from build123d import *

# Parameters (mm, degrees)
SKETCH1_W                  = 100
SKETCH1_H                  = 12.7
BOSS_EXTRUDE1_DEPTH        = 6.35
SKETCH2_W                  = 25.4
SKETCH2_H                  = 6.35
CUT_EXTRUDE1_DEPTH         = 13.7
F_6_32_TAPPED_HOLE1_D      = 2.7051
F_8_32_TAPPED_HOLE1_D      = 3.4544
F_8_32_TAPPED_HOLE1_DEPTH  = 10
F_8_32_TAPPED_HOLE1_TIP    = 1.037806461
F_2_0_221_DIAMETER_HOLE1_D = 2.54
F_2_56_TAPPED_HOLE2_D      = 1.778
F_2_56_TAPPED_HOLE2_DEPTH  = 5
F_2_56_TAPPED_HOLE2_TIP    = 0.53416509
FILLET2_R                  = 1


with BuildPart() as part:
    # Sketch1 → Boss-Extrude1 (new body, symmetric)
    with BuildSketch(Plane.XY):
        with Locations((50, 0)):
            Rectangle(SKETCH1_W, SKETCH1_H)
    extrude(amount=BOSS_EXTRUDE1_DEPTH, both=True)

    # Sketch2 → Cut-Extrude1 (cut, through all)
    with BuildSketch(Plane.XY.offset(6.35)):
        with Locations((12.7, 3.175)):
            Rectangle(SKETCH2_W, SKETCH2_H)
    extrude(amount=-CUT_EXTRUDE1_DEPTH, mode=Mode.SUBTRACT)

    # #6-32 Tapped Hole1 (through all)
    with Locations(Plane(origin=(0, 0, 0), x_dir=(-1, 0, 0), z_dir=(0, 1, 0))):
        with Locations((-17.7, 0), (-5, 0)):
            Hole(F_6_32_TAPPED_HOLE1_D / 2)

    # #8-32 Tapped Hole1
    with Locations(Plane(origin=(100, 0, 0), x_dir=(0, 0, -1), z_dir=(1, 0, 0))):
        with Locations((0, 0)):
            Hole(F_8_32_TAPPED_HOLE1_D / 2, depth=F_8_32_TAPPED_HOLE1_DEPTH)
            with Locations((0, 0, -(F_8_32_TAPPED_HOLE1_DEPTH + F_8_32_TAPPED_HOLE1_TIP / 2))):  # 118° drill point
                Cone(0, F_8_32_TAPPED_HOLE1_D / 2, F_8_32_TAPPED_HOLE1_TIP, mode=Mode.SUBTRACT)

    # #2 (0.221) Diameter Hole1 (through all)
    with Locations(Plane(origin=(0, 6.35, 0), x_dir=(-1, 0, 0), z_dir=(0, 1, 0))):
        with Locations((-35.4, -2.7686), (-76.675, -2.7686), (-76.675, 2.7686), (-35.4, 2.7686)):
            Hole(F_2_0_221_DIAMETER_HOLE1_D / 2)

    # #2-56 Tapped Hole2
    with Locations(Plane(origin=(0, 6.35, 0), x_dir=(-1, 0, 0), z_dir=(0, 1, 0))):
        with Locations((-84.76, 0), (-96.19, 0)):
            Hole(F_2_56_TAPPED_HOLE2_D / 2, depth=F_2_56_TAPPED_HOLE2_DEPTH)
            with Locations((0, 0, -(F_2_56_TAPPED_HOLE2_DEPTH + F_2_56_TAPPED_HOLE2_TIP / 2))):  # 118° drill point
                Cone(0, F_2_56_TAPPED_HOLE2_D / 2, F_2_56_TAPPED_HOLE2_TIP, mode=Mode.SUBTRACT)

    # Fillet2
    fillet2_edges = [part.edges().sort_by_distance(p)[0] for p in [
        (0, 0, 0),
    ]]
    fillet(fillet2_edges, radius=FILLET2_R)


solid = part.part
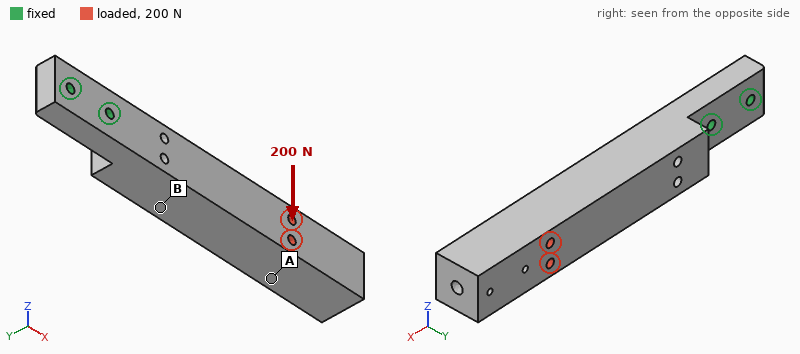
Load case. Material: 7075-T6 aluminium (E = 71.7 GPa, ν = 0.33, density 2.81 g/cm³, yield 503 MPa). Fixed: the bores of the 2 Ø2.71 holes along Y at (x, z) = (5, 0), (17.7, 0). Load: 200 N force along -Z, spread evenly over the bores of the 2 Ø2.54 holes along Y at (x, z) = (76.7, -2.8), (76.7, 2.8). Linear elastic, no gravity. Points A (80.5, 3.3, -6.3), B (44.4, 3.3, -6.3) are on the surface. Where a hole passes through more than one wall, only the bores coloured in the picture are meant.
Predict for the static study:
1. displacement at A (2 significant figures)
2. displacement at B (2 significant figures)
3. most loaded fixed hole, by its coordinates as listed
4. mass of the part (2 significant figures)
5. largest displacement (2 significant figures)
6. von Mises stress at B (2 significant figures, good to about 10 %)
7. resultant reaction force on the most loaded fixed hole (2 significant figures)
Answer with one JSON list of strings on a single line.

["0.21 mm", "0.069 mm", "(17.7, 0)", "38 g", "0.28 mm", "19 MPa", "840 N"]
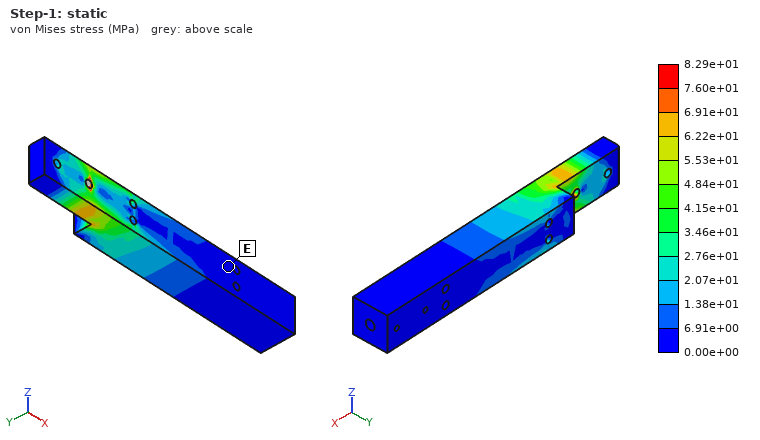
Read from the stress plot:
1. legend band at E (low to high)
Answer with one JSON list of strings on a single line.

["0.00e+00 to 6.91e+00 MPa"]
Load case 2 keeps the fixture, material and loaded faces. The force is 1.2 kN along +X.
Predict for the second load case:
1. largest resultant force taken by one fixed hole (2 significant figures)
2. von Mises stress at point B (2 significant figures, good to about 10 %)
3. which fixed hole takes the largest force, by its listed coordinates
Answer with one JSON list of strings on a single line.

["1.0 kN", "7.6 MPa", "(17.7, 0)"]
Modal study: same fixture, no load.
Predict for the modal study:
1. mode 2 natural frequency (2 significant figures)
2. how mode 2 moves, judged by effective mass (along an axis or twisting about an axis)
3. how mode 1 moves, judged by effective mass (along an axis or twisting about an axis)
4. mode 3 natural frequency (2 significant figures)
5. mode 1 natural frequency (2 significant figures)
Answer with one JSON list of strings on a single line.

["1100 Hz", "along Z", "along Y", "6000 Hz", "750 Hz"]
